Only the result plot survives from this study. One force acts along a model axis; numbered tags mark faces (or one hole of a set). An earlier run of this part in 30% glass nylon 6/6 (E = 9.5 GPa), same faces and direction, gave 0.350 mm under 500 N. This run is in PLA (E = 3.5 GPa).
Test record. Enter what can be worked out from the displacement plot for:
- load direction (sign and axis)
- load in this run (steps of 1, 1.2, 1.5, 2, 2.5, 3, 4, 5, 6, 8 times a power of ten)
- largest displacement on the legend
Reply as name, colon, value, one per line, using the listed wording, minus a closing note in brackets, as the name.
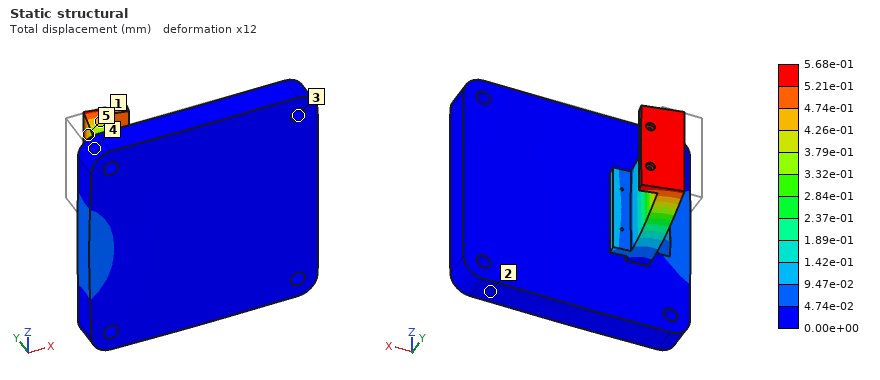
load direction: +X
load in this run: 300 N
largest displacement on the legend: 5.68e-01 mm
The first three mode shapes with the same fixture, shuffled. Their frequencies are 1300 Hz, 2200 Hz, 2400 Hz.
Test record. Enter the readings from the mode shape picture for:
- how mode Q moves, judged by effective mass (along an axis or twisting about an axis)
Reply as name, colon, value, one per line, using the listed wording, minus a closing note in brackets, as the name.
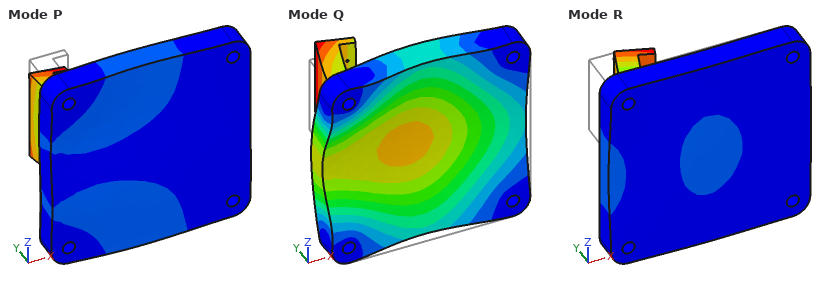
how mode Q moves, judged by effective mass: along Y
